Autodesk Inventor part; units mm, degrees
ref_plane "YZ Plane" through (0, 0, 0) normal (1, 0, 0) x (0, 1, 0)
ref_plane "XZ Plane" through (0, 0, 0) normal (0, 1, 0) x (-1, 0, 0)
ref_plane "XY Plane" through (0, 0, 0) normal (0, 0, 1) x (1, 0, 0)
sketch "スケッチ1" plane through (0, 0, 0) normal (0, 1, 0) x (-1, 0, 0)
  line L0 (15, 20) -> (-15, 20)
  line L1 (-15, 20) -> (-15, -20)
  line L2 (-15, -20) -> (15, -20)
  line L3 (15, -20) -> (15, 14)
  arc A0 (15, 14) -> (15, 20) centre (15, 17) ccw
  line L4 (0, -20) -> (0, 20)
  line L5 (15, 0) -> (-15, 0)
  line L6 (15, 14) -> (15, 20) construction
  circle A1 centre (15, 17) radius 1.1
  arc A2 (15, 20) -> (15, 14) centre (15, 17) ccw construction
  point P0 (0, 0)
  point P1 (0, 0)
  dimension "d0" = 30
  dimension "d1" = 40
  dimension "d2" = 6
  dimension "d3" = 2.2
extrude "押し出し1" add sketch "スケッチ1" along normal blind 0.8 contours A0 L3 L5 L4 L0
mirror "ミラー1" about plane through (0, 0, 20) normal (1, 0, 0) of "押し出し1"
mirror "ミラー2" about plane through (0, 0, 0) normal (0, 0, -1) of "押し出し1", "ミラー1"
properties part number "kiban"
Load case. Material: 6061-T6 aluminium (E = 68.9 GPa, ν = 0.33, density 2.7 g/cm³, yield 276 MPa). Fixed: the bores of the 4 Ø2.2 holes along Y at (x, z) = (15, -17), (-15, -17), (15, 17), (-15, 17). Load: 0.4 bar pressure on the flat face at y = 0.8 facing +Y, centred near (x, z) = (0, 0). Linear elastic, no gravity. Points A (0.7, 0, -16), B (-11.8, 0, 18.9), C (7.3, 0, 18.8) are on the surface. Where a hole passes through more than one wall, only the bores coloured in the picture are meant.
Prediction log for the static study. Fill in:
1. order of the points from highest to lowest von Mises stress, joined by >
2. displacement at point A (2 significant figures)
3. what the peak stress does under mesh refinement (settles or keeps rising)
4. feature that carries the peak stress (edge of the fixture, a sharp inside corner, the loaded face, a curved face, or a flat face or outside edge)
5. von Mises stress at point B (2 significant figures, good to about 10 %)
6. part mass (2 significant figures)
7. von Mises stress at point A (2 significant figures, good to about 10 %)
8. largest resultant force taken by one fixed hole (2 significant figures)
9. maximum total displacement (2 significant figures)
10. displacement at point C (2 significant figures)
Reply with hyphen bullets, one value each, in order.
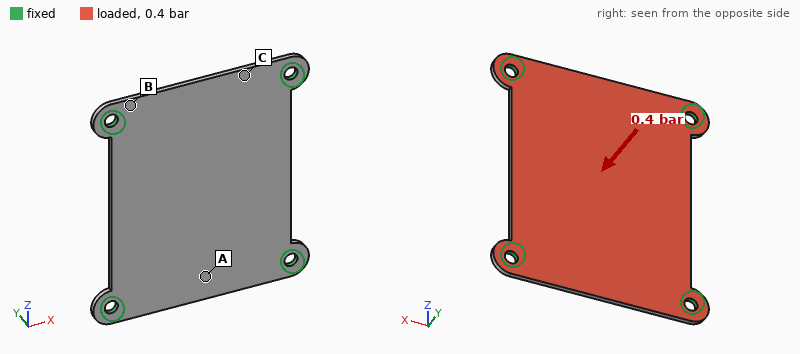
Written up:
- B > A > C
- 43 µm
- keeps rising
- edge of the fixture
- 32 MPa
- 2.7 g
- 18 MPa
- 12 N
- 96 µm
- 16 µm
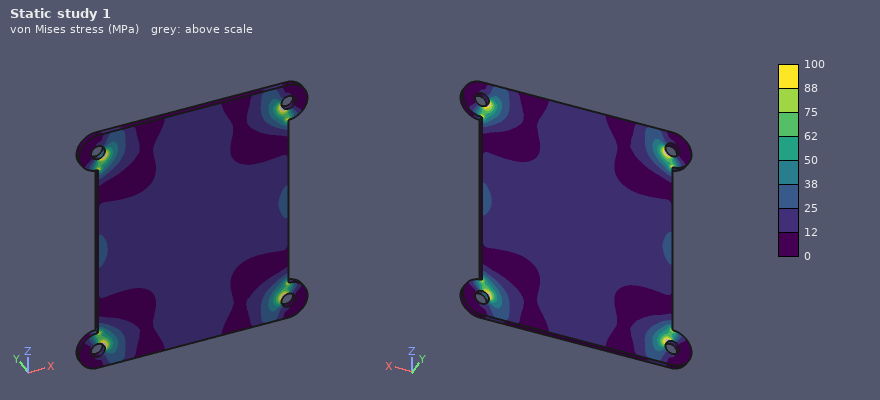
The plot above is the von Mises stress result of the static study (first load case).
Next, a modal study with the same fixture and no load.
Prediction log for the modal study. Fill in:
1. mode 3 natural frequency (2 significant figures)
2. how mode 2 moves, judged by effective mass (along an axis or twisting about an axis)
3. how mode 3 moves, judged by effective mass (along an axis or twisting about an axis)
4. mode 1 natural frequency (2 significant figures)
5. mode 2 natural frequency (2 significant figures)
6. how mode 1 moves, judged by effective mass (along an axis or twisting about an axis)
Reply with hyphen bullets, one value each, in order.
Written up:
- 5100 Hz
- twisting about Z
- twisting about X
- 2600 Hz
- 4600 Hz
- along Y
